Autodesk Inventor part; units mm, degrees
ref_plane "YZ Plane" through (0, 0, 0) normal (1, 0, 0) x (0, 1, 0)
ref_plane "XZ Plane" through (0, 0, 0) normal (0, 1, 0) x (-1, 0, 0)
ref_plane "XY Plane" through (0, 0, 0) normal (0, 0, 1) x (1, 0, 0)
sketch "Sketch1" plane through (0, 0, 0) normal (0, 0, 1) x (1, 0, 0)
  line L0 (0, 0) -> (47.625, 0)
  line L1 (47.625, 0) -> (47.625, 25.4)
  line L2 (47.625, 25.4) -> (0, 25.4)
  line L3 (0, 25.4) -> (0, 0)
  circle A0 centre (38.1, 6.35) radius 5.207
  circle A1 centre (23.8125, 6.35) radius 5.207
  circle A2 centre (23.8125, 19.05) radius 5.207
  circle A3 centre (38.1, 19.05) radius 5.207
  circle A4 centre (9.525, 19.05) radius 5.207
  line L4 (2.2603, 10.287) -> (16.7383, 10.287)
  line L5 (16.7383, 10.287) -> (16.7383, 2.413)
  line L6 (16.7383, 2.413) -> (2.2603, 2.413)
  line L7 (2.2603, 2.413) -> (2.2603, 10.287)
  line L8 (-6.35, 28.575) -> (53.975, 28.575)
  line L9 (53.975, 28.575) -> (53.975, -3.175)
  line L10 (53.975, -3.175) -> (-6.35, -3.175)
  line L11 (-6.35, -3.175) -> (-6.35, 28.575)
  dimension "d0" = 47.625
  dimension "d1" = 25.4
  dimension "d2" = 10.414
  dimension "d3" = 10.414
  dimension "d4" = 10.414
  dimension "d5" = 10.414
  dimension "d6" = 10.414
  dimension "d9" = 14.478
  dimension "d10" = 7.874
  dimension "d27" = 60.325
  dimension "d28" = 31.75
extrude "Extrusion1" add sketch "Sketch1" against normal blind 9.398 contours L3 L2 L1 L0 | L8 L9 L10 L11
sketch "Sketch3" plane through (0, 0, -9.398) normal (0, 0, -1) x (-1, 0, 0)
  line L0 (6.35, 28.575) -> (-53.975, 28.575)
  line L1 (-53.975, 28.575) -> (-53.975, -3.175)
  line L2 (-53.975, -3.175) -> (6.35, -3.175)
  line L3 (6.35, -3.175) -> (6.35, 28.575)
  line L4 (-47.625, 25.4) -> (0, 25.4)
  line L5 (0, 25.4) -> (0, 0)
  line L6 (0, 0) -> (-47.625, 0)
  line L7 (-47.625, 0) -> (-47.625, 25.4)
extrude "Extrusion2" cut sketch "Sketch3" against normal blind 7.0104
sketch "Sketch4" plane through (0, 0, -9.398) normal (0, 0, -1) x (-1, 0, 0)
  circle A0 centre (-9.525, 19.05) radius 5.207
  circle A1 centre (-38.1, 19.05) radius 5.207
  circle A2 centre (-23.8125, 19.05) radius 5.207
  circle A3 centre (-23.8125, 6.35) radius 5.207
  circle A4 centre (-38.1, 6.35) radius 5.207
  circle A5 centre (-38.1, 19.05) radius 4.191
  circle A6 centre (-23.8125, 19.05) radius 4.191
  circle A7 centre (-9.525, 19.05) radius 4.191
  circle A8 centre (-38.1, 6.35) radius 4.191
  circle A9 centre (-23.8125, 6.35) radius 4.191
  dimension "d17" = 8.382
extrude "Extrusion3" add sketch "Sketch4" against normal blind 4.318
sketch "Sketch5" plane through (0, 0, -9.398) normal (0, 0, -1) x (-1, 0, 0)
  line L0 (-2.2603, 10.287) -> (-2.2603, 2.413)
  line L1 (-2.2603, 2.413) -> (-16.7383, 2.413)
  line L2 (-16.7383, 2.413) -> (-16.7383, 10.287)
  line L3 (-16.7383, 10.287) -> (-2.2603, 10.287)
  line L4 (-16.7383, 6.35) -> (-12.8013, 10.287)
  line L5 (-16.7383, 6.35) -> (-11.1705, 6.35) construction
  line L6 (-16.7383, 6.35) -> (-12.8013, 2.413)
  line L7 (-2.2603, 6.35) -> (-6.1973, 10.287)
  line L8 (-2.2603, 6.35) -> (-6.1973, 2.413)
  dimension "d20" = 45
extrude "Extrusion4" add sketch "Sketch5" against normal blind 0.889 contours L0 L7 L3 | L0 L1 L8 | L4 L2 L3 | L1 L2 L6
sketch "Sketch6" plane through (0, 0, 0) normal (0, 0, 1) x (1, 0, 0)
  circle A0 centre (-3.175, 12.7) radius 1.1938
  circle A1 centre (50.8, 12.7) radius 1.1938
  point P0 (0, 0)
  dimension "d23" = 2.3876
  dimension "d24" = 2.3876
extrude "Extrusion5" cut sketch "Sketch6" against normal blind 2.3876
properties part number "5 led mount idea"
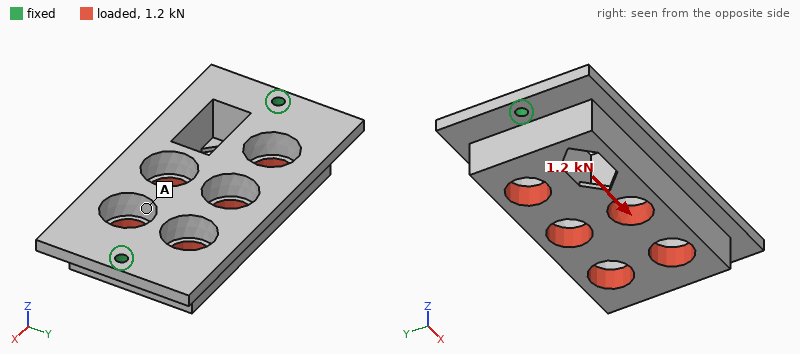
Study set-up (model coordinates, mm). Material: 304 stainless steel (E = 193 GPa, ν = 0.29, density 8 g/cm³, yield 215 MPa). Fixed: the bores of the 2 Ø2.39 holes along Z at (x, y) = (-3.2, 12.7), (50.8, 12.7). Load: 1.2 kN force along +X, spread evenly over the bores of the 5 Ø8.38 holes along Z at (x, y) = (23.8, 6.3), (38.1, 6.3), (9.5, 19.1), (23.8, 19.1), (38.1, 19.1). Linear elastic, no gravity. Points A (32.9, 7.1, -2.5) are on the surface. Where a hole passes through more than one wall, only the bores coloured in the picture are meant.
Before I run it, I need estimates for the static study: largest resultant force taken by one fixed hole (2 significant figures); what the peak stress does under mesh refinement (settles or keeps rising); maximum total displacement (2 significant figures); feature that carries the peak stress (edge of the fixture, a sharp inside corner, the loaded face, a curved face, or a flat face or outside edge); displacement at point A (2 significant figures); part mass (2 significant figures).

630 N
keeps rising
2.6 µm
edge of the fixture
2.2 µm
69 g
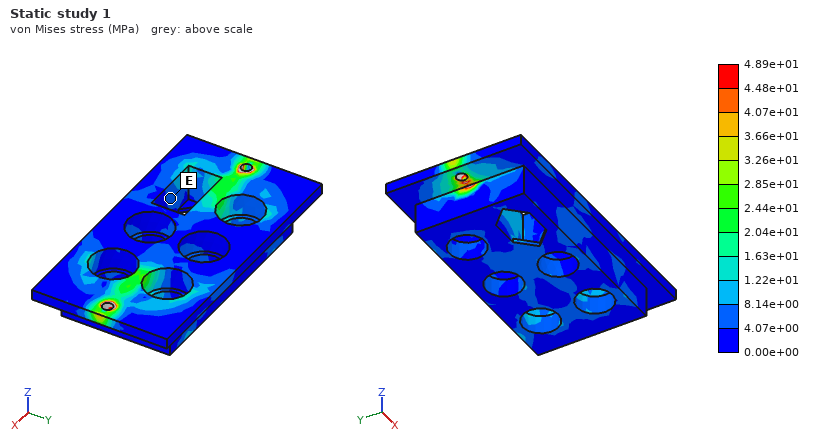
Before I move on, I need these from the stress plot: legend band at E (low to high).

4.07e+00 to 8.14e+00 MPa
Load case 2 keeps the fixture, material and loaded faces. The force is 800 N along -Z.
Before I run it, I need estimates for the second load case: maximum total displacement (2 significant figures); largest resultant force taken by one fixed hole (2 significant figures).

16 µm
650 N
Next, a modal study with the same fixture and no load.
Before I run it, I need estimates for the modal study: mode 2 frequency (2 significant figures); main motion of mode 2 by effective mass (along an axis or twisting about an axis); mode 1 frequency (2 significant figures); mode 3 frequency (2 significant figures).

7000 Hz
along Z
3200 Hz
10 kHz
